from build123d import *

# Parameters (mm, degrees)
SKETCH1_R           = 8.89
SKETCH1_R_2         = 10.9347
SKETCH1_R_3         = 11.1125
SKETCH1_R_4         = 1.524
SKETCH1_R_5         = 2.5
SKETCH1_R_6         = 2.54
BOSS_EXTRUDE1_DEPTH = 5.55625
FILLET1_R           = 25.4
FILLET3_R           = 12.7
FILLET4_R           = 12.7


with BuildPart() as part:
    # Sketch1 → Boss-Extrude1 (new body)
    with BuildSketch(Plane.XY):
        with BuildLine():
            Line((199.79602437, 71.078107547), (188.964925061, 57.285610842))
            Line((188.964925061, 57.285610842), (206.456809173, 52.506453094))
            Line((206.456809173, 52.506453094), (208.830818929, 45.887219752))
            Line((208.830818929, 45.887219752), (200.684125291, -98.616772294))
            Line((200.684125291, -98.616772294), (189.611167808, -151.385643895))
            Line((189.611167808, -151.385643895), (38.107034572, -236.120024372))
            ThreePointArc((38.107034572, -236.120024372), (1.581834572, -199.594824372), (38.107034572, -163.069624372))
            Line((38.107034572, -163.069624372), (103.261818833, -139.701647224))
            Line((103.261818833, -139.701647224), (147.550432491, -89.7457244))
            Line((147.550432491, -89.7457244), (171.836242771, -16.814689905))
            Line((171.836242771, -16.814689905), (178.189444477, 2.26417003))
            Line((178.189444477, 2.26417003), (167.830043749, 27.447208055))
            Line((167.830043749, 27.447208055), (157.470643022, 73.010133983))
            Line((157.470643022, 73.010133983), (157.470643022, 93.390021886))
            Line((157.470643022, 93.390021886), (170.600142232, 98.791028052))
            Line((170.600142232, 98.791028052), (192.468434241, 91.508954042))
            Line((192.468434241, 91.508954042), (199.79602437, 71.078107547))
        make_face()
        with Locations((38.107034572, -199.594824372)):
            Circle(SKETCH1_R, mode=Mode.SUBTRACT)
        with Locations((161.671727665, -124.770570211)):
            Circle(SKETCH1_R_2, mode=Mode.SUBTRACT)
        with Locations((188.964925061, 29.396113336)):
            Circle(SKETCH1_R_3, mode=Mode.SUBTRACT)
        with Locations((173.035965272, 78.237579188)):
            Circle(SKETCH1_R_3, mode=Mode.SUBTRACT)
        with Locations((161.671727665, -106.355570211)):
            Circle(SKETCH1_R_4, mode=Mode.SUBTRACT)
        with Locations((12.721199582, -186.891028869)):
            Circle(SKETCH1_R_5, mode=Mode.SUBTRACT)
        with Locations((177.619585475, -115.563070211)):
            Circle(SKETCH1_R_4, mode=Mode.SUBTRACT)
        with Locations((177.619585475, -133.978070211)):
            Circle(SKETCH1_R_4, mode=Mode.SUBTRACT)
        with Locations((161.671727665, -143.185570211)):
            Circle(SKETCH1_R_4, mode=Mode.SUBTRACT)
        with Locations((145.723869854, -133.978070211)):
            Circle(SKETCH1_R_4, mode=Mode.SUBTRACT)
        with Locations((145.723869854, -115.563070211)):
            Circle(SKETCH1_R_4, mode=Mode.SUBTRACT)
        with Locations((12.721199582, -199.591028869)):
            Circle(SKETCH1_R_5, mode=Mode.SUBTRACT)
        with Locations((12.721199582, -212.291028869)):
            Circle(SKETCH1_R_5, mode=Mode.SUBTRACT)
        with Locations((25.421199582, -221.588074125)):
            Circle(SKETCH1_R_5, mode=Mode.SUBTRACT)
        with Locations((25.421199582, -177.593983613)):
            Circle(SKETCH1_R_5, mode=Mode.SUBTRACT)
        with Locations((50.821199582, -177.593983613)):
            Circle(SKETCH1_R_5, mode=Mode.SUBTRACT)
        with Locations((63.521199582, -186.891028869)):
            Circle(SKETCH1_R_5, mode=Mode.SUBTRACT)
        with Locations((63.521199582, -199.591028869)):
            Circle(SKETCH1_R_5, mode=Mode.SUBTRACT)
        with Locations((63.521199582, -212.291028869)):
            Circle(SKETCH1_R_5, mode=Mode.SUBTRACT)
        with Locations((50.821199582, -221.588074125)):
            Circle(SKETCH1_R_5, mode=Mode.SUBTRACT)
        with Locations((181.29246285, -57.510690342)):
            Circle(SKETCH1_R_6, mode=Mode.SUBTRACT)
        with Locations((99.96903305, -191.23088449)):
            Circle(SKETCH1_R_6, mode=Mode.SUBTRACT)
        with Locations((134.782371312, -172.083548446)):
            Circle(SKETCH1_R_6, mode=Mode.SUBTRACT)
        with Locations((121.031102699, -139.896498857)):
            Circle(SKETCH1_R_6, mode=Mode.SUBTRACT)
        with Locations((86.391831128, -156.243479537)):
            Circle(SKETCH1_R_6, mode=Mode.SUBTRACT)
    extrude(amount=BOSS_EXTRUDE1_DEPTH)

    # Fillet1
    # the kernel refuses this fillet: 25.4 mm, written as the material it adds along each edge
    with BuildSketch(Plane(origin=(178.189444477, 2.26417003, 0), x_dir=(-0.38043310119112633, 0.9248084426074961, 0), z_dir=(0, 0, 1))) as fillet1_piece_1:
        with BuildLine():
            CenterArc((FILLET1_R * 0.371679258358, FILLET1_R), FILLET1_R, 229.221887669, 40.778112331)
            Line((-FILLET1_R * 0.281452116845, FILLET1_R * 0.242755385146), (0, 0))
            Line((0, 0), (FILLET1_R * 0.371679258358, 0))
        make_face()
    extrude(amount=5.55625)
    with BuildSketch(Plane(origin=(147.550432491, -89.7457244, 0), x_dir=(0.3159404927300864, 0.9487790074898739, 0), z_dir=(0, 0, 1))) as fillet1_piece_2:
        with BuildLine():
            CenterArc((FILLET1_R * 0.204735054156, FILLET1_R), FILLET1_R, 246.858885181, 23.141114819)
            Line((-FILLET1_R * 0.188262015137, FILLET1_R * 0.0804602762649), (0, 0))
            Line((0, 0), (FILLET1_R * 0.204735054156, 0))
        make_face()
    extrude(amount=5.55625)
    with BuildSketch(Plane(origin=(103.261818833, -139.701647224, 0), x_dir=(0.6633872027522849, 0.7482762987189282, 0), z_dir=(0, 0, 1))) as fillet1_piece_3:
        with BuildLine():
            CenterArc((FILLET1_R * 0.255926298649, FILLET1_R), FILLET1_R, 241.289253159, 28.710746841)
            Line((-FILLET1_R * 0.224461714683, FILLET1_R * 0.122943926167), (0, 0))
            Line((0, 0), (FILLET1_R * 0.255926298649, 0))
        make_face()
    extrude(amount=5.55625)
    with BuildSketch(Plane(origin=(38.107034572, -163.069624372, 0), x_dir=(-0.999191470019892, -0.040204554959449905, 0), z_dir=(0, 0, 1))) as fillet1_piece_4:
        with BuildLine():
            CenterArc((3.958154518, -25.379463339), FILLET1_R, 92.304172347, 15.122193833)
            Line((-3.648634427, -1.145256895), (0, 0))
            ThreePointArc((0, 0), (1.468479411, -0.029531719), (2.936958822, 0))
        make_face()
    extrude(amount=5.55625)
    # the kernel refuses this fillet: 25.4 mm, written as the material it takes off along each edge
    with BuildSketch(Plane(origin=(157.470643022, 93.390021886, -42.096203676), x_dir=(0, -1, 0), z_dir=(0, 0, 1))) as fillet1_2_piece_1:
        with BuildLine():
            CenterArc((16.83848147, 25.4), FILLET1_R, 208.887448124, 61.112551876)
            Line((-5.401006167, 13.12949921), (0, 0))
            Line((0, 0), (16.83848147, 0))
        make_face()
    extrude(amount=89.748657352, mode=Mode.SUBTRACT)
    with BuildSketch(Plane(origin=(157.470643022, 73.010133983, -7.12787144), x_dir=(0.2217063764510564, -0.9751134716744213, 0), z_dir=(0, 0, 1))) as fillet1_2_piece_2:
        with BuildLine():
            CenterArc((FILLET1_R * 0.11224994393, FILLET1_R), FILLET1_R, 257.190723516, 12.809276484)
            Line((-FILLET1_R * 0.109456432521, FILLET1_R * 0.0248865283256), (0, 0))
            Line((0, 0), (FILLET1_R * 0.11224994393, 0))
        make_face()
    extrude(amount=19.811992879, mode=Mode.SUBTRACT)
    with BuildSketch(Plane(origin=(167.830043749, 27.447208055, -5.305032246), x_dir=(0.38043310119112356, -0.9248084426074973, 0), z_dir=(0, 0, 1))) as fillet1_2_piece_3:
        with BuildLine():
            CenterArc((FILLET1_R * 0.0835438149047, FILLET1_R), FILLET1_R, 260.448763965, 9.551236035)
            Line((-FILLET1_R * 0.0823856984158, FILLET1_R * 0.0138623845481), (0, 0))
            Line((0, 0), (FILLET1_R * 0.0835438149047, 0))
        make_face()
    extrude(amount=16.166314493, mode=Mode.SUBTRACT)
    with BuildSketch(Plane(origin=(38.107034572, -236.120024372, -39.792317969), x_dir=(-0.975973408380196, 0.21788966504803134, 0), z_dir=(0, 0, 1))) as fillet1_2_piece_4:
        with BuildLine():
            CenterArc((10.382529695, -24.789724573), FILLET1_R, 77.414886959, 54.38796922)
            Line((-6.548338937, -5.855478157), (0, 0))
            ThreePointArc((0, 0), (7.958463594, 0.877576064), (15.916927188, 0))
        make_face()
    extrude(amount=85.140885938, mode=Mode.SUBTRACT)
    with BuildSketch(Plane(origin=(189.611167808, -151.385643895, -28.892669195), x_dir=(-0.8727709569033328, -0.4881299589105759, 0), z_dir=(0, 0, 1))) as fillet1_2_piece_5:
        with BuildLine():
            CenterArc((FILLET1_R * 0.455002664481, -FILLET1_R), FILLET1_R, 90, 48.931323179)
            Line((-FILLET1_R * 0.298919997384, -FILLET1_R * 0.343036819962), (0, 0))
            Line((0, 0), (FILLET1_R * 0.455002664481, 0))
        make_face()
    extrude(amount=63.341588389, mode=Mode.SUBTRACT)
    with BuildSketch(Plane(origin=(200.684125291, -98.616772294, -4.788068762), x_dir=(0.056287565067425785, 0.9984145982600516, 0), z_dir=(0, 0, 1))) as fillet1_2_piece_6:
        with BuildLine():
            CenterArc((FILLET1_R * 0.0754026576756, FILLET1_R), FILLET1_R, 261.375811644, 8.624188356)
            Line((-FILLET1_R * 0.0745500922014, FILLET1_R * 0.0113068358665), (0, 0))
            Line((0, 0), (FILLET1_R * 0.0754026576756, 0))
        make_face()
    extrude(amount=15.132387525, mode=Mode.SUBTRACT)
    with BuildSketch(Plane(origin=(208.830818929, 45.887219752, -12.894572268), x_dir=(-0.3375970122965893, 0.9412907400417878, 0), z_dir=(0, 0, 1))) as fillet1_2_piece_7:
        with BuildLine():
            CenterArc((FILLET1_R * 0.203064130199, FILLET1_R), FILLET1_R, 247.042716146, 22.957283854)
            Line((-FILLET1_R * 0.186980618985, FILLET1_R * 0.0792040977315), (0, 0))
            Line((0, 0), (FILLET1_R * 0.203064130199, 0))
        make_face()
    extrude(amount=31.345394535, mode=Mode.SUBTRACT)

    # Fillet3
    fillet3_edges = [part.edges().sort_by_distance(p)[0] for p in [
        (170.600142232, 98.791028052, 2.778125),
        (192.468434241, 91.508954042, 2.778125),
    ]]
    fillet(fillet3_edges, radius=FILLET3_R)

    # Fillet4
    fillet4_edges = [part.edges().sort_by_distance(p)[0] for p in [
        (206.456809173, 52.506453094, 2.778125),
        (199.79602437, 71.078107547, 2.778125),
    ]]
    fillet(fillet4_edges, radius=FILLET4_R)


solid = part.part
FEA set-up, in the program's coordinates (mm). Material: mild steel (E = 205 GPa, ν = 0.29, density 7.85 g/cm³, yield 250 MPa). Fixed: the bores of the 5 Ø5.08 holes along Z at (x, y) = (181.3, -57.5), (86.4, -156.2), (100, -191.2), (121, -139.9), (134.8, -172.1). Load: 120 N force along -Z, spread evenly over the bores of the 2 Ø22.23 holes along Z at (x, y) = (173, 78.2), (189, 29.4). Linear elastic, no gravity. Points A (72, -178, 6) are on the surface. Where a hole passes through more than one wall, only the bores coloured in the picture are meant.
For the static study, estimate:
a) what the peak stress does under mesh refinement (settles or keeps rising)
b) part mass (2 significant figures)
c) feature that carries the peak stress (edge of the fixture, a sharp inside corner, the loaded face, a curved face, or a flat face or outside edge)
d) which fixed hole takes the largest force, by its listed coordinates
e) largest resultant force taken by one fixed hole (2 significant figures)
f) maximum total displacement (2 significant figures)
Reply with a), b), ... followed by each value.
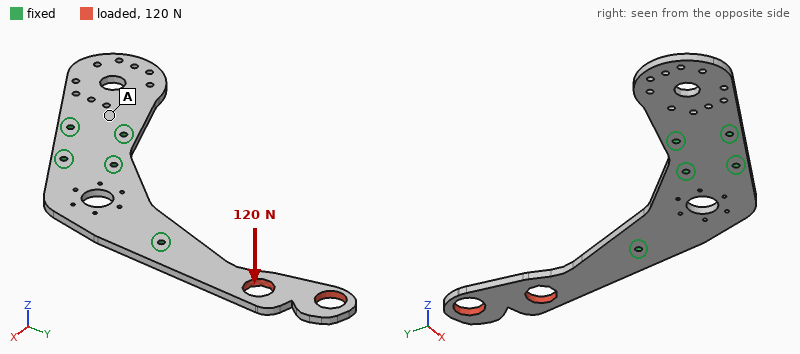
a) keeps rising
b) 810 g
c) edge of the fixture
d) (181.3, -57.5)
e) 140 N
f) 0.94 mm
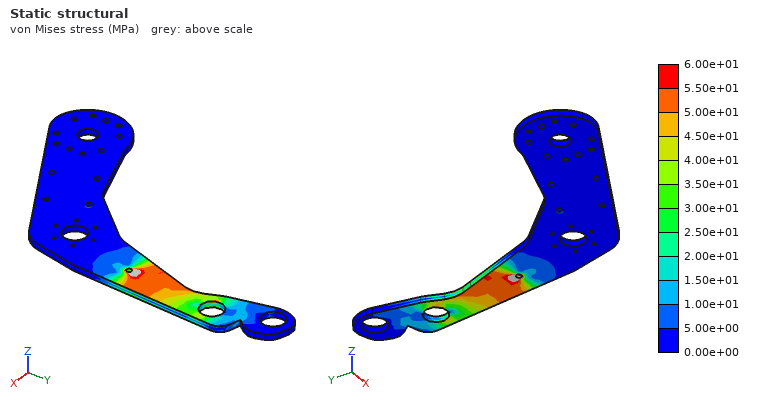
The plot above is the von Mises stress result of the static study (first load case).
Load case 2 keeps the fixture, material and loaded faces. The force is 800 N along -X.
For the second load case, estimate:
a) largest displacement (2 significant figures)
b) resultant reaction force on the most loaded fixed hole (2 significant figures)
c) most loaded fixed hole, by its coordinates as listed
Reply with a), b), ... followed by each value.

a) 0.21 mm
b) 1.8 kN
c) (181.3, -57.5)
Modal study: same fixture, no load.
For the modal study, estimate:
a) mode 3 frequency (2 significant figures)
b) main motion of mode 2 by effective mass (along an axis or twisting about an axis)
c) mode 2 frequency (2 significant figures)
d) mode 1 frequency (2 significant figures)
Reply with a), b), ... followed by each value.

a) 1100 Hz
b) along Z
c) 530 Hz
d) 220 Hz
